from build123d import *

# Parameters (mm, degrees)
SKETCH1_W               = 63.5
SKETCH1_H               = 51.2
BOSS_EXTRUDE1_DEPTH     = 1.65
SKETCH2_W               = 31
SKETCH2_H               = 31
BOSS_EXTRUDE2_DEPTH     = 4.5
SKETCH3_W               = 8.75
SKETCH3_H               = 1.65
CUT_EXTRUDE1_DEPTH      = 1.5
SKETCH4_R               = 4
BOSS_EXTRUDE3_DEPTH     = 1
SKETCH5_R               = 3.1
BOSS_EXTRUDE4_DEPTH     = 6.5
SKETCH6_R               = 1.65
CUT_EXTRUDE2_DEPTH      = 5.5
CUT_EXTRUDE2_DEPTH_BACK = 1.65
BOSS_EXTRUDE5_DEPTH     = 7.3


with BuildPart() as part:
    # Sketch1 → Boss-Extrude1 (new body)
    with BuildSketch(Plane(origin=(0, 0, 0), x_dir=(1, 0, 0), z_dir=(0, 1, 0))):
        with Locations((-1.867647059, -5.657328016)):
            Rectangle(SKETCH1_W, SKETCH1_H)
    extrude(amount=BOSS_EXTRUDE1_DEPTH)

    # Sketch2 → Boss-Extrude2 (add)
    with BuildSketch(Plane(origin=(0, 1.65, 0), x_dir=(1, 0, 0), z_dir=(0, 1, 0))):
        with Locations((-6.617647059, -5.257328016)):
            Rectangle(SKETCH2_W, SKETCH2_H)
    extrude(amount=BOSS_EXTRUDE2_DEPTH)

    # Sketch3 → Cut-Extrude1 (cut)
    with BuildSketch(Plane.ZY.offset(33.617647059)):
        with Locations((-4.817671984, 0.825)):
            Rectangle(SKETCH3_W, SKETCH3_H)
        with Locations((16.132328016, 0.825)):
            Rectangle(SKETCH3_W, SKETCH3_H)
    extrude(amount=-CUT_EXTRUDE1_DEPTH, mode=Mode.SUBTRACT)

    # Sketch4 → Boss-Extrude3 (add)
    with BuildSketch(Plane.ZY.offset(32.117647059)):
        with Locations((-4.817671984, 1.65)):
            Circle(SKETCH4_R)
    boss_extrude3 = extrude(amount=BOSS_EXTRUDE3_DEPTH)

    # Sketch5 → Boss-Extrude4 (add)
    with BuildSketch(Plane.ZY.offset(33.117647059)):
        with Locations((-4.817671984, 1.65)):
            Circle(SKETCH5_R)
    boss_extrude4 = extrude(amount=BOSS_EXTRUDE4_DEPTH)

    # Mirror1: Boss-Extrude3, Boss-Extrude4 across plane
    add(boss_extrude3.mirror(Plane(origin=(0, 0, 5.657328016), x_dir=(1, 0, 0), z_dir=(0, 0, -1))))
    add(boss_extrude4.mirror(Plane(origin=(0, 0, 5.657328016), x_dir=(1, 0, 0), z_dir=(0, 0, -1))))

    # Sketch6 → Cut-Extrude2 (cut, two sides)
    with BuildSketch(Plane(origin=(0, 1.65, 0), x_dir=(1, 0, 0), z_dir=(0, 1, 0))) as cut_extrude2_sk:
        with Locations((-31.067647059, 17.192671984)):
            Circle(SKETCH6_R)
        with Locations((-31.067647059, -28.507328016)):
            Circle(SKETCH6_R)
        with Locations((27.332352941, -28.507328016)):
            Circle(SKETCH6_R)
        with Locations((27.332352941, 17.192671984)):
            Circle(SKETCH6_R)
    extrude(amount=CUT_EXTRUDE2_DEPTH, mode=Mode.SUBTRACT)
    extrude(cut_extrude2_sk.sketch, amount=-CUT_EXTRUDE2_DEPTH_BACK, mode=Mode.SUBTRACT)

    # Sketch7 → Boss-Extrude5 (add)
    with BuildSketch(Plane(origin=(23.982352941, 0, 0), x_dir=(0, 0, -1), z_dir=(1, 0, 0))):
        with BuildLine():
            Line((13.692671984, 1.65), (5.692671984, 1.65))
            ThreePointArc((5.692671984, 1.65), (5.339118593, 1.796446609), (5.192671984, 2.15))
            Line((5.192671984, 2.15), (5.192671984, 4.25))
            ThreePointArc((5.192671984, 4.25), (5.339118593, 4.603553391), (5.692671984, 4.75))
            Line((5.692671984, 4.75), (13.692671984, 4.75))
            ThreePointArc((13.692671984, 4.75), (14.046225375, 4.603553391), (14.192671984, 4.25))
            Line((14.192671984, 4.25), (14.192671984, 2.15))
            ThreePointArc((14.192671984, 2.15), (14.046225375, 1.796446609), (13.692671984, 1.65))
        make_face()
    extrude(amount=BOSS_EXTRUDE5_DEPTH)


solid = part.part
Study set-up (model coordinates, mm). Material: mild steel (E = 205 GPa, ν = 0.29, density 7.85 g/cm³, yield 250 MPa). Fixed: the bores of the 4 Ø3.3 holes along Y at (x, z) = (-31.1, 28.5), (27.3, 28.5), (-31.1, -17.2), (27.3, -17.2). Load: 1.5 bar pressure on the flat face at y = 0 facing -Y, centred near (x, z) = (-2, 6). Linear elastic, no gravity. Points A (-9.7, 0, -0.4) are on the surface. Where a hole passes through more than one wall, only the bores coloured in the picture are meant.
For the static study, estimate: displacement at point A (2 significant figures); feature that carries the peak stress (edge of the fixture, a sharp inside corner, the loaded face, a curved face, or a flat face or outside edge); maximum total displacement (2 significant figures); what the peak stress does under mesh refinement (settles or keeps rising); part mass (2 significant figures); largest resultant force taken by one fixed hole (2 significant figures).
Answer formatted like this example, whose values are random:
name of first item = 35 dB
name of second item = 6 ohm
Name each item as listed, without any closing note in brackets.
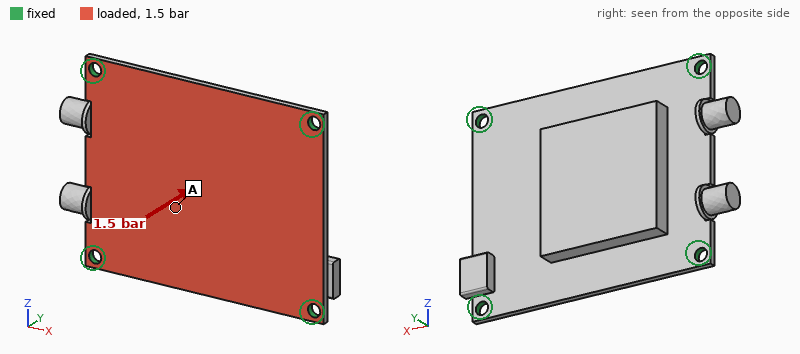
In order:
displacement at point A = 31 µm
feature that carries the peak stress = edge of the fixture
maximum total displacement = 44 µm
what the peak stress does under mesh refinement = keeps rising
part mass = 81 g
largest resultant force taken by one fixed hole = 140 N
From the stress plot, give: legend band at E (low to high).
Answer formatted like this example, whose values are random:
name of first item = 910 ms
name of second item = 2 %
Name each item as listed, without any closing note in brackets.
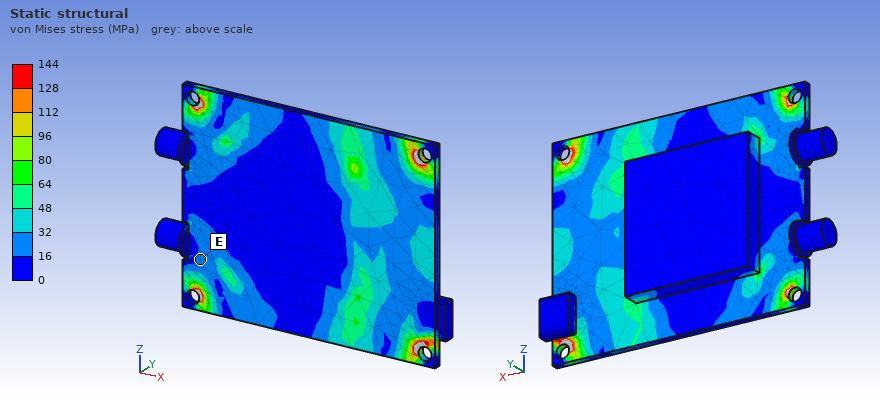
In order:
legend band at E = 16 to 32 MPa
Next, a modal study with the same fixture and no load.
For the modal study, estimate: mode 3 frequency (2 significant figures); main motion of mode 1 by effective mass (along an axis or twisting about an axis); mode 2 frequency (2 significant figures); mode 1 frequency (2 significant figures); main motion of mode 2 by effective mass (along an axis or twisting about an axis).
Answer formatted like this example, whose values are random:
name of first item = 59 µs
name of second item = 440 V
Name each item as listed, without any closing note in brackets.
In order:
mode 3 frequency = 4100 Hz
main motion of mode 1 by effective mass = along Y
mode 2 frequency = 3900 Hz
mode 1 frequency = 2100 Hz
main motion of mode 2 by effective mass = twisting about X
